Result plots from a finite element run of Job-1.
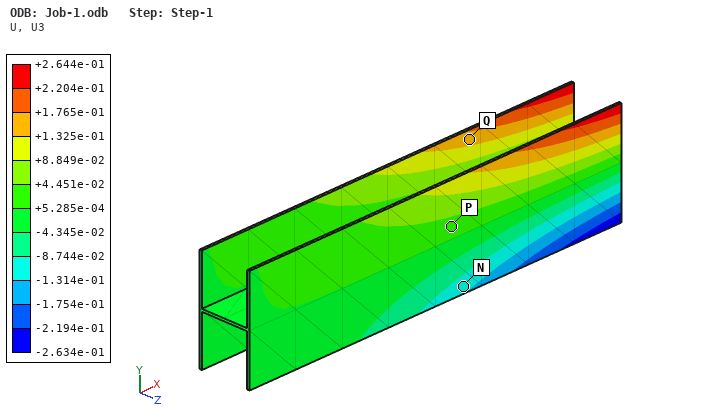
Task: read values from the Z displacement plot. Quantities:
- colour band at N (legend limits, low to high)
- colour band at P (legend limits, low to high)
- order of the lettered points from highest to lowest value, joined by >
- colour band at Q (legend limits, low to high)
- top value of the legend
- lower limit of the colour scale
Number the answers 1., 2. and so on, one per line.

1. -1.314e-01 to -8.744e-02
2. +5.285e-04 to +4.451e-02
3. Q > P > N
4. +1.325e-01 to +1.765e-01
5. +2.644e-01
6. -2.634e-01
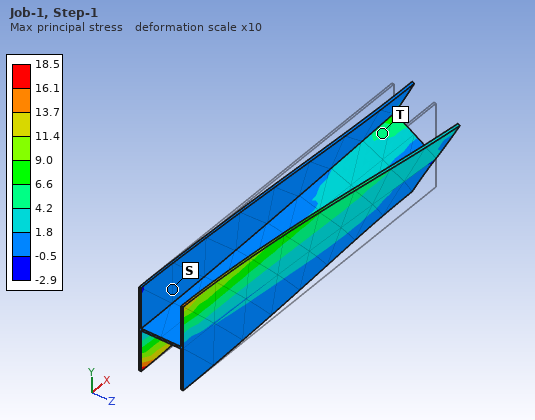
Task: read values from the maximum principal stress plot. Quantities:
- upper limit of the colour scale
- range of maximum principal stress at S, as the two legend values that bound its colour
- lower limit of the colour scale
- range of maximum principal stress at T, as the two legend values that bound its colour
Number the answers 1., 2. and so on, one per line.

1. 18.5
2. -0.5 to 1.8
3. -2.9
4. 4.2 to 6.6
